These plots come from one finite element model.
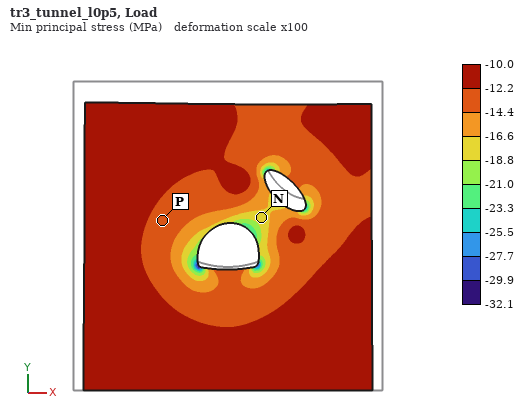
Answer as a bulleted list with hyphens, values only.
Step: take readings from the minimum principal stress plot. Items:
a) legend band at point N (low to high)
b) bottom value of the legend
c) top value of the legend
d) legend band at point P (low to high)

- -18.8 to -16.6 MPa
- -32.1 MPa
- -10.0 MPa
- -14.4 to -12.2 MPa
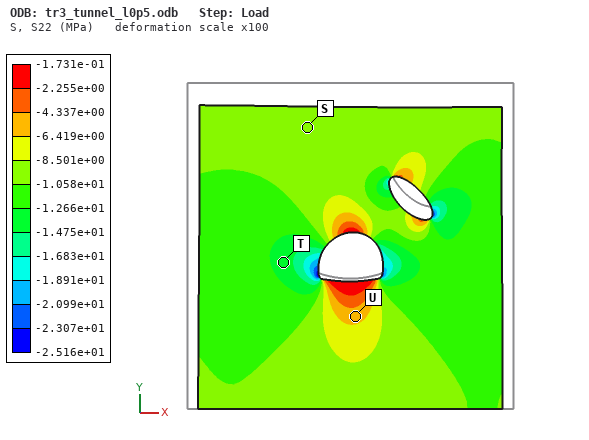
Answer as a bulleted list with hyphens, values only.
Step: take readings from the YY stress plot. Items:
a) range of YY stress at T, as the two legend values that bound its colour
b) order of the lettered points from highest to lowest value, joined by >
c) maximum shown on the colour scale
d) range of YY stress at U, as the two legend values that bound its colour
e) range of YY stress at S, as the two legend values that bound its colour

- -1.475e+01 to -1.266e+01 MPa
- U > S > T
- -1.731e-01 MPa
- -6.419e+00 to -4.337e+00 MPa
- -1.058e+01 to -8.501e+00 MPa
